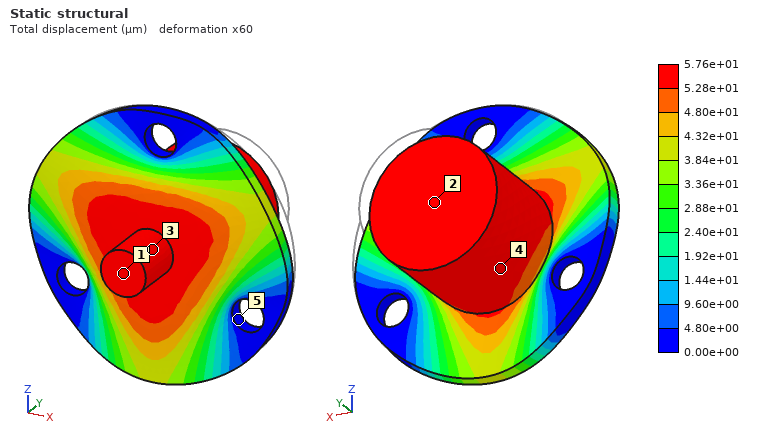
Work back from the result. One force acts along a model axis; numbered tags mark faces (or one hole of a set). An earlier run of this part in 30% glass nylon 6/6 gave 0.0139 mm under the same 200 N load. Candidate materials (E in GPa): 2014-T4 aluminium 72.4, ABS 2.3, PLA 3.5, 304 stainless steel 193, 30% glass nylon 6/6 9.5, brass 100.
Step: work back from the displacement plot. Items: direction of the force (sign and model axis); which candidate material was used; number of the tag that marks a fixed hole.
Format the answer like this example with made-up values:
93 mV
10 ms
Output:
-Y
ABS
5
